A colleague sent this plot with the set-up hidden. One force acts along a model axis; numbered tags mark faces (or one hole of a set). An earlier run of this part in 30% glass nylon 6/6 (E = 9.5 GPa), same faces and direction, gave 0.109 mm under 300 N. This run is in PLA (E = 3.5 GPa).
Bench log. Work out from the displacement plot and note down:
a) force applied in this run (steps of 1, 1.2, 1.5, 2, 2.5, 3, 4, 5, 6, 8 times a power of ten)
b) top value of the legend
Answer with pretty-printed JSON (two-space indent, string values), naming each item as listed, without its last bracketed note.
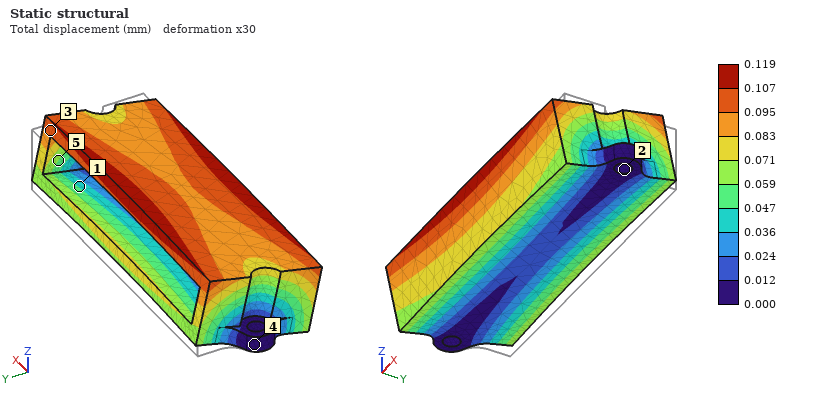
{
  "force applied in this run": "120 N",
  "top value of the legend": "0.119 mm"
}
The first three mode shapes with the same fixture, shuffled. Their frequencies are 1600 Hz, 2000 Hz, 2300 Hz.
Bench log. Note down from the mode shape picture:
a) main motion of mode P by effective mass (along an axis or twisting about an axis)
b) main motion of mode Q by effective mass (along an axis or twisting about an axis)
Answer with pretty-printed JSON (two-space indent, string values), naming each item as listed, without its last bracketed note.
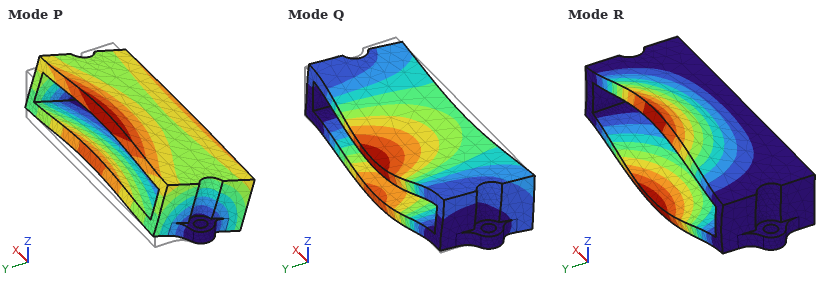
{
  "main motion of mode P by effective mass": "along Y",
  "main motion of mode Q by effective mass": "along Z"
}
